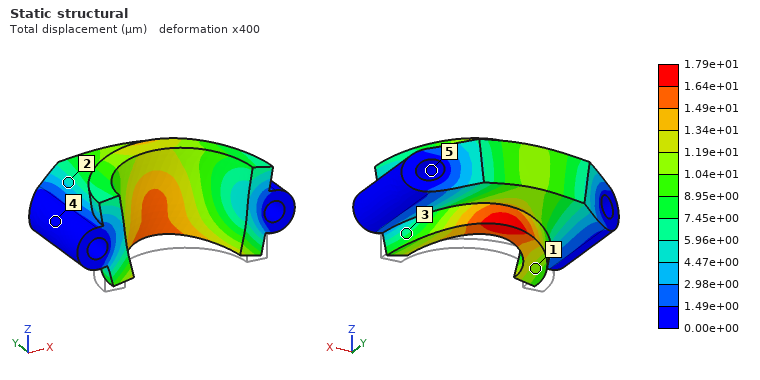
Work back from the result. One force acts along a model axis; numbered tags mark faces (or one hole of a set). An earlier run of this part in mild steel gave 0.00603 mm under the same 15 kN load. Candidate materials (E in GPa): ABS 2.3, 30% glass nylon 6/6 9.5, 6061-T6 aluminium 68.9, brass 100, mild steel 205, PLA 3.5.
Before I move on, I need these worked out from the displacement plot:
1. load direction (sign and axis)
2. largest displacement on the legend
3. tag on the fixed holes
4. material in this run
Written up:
+Z
1.79e+01 µm
5
6061-T6 aluminium
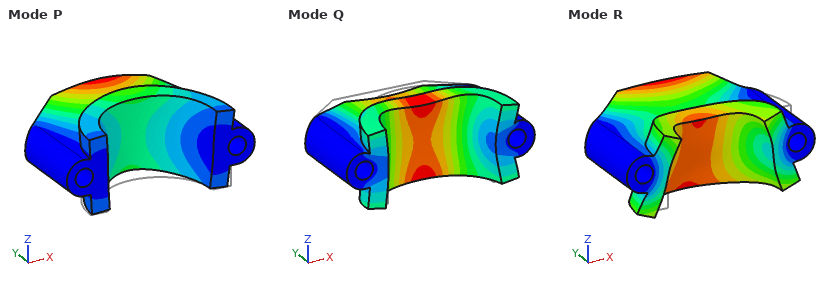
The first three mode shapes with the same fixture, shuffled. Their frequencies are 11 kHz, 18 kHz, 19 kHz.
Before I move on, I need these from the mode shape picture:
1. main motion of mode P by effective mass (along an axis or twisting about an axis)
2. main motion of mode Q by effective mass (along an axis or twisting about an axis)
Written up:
along Z
along Y
